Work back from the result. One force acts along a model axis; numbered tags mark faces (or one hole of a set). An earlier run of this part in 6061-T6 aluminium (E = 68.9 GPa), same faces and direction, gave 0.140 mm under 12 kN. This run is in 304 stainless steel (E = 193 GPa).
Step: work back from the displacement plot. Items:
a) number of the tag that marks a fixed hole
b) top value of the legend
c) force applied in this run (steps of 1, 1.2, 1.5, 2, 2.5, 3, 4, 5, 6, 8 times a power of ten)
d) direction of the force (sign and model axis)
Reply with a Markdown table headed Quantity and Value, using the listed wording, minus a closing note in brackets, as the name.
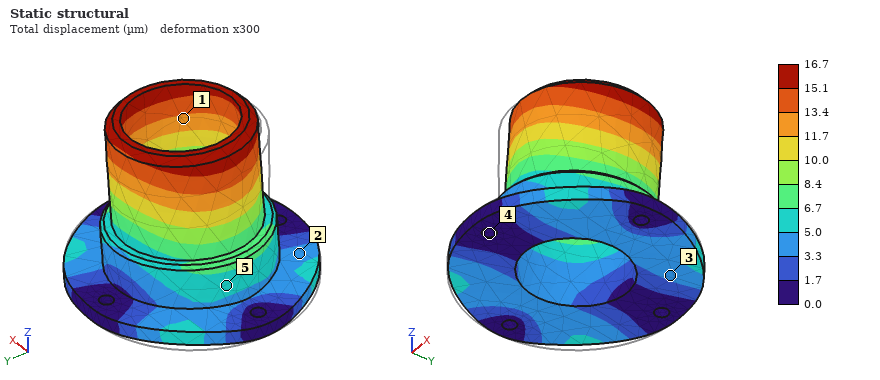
| Quantity | Value |
|---|---|
| number of the tag that marks a fixed hole | 4 |
| top value of the legend | 16.7 µm |
| force applied in this run | 4 kN |
| direction of the force | +X |
